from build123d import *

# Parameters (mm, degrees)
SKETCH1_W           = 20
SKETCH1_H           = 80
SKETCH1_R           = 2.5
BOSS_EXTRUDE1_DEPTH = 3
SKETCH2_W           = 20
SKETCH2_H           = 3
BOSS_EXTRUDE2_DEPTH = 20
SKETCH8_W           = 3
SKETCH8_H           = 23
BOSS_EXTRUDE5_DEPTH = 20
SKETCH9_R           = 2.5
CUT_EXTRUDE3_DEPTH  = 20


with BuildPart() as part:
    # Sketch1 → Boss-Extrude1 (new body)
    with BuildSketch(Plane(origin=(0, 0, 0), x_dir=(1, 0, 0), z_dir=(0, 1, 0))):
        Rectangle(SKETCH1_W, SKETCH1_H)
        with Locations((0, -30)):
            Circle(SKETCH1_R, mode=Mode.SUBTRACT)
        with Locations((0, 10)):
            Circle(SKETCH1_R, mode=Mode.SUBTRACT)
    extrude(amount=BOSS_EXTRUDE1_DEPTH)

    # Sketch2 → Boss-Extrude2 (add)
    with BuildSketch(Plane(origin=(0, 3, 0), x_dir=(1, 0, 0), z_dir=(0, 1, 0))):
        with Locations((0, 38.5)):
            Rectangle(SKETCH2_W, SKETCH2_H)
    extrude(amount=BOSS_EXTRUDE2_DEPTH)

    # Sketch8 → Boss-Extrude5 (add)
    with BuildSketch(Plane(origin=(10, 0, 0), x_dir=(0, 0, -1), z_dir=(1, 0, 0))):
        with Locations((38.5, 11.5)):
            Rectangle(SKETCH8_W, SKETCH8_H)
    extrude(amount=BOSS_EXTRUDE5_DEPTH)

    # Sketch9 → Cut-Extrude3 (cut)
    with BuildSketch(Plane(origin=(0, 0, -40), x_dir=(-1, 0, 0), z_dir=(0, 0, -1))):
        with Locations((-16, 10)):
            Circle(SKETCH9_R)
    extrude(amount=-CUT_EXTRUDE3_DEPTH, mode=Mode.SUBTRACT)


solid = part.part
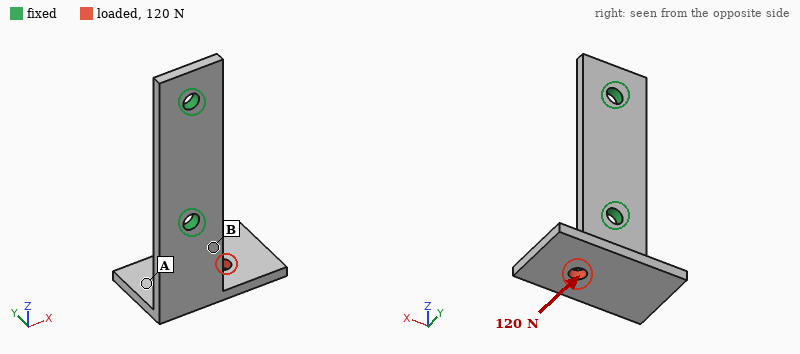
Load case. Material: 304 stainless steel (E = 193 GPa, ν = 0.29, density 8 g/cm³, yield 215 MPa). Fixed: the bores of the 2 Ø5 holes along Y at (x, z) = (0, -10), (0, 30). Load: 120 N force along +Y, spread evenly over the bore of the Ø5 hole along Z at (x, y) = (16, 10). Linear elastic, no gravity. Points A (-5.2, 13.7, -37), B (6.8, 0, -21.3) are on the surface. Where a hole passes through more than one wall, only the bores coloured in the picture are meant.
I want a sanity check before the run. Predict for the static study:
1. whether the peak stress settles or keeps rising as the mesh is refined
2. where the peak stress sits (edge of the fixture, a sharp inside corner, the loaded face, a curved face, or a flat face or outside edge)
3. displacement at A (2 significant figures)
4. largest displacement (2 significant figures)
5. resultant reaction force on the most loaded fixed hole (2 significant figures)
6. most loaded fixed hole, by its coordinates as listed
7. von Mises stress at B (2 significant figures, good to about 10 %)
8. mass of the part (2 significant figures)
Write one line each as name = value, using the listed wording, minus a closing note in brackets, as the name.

whether the peak stress settles or keeps rising as the mesh is refined = keeps rising
where the peak stress sits = edge of the fixture
displacement at A = 0.10 mm
largest displacement = 0.26 mm
resultant reaction force on the most loaded fixed hole = 120 N
most loaded fixed hole, by its coordinates as listed = (0, -10)
von Mises stress at B = 85 MPa
mass of the part = 58 g
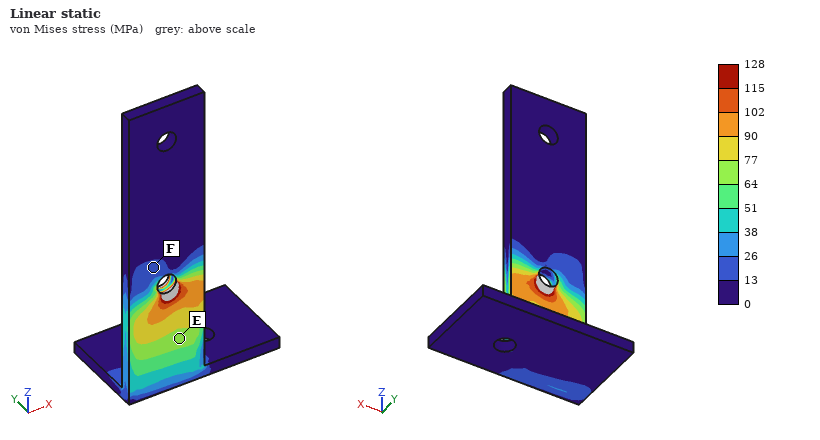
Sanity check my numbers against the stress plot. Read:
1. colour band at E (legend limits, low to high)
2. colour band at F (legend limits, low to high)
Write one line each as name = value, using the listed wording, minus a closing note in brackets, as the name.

colour band at E = 64 to 77 MPa
colour band at F = 13 to 26 MPa
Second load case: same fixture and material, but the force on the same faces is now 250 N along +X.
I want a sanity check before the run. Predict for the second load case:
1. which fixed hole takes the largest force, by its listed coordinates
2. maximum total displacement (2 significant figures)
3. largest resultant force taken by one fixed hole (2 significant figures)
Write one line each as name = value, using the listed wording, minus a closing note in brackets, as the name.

which fixed hole takes the largest force, by its listed coordinates = (0, -10)
maximum total displacement = 0.16 mm
largest resultant force taken by one fixed hole = 360 N
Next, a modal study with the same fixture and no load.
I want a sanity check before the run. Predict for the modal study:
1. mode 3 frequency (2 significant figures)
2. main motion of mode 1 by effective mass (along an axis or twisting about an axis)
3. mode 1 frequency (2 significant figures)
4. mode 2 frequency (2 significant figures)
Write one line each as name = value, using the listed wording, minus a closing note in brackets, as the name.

mode 3 frequency = 2600 Hz
main motion of mode 1 by effective mass = along Y
mode 1 frequency = 880 Hz
mode 2 frequency = 1400 Hz
